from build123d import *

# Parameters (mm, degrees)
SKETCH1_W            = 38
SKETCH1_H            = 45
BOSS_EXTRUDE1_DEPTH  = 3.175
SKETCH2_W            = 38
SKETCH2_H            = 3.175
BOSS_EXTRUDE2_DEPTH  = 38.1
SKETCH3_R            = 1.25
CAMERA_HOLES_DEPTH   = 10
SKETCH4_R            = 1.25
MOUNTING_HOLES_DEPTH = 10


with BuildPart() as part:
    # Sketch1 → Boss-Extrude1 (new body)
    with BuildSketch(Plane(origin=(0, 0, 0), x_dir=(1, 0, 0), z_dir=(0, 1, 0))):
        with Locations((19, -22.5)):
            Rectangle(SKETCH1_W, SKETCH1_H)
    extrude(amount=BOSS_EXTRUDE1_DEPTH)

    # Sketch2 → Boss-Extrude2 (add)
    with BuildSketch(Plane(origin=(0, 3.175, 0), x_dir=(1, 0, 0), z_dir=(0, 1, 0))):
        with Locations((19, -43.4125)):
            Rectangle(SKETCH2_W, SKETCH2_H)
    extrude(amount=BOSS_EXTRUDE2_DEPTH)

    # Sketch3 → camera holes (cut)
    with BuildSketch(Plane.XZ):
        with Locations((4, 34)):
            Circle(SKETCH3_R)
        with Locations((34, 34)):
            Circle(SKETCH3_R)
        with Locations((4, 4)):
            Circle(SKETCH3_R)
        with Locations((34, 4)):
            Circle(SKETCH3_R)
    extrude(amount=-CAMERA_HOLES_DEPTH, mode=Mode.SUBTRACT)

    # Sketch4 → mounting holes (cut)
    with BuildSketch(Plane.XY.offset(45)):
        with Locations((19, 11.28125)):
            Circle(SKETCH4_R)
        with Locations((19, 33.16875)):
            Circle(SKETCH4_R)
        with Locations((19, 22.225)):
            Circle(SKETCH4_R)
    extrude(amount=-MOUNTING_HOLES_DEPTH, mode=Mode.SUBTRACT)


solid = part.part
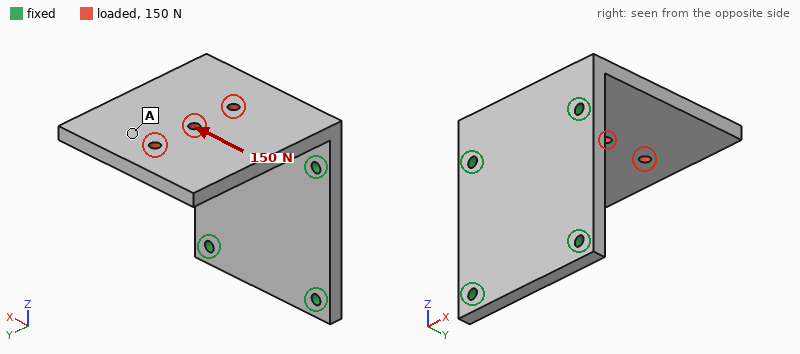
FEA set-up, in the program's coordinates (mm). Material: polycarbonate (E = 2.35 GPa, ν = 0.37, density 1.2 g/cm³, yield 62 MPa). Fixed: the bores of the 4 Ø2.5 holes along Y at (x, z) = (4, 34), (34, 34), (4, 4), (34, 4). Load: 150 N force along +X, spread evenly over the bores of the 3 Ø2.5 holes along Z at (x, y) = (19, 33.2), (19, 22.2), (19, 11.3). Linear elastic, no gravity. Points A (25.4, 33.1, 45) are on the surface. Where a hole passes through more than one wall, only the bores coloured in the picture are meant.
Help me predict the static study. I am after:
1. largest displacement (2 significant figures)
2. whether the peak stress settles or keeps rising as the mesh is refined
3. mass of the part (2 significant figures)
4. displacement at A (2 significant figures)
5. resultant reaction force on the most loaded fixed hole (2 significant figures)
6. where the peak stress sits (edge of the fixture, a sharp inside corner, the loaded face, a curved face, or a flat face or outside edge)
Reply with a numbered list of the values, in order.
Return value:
1. 0.84 mm
2. keeps rising
3. 12 g
4. 0.54 mm
5. 140 N
6. edge of the fixture
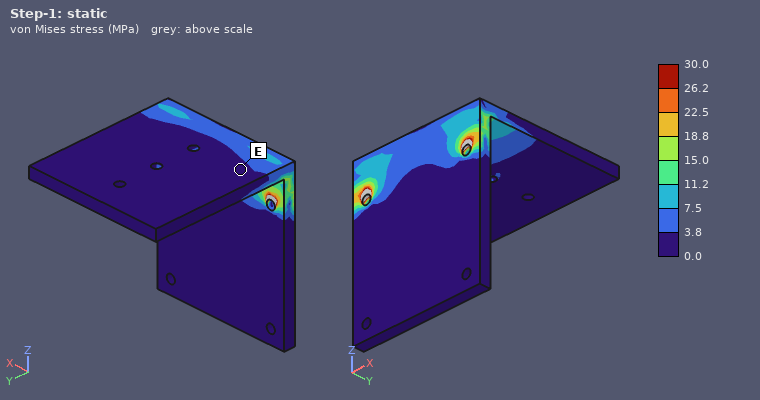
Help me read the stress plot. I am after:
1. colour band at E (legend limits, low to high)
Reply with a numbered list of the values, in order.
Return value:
1. 0.0 to 3.8 MPa
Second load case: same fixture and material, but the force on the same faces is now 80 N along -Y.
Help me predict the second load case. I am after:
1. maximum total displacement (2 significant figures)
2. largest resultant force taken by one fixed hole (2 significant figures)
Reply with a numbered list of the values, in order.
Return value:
1. 0.72 mm
2. 43 N
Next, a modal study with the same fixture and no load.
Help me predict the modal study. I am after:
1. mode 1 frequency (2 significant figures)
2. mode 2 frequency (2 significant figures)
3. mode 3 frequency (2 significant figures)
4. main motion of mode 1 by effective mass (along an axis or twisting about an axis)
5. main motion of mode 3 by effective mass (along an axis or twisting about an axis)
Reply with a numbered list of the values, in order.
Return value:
1. 340 Hz
2. 920 Hz
3. 1300 Hz
4. along Z
5. along X
